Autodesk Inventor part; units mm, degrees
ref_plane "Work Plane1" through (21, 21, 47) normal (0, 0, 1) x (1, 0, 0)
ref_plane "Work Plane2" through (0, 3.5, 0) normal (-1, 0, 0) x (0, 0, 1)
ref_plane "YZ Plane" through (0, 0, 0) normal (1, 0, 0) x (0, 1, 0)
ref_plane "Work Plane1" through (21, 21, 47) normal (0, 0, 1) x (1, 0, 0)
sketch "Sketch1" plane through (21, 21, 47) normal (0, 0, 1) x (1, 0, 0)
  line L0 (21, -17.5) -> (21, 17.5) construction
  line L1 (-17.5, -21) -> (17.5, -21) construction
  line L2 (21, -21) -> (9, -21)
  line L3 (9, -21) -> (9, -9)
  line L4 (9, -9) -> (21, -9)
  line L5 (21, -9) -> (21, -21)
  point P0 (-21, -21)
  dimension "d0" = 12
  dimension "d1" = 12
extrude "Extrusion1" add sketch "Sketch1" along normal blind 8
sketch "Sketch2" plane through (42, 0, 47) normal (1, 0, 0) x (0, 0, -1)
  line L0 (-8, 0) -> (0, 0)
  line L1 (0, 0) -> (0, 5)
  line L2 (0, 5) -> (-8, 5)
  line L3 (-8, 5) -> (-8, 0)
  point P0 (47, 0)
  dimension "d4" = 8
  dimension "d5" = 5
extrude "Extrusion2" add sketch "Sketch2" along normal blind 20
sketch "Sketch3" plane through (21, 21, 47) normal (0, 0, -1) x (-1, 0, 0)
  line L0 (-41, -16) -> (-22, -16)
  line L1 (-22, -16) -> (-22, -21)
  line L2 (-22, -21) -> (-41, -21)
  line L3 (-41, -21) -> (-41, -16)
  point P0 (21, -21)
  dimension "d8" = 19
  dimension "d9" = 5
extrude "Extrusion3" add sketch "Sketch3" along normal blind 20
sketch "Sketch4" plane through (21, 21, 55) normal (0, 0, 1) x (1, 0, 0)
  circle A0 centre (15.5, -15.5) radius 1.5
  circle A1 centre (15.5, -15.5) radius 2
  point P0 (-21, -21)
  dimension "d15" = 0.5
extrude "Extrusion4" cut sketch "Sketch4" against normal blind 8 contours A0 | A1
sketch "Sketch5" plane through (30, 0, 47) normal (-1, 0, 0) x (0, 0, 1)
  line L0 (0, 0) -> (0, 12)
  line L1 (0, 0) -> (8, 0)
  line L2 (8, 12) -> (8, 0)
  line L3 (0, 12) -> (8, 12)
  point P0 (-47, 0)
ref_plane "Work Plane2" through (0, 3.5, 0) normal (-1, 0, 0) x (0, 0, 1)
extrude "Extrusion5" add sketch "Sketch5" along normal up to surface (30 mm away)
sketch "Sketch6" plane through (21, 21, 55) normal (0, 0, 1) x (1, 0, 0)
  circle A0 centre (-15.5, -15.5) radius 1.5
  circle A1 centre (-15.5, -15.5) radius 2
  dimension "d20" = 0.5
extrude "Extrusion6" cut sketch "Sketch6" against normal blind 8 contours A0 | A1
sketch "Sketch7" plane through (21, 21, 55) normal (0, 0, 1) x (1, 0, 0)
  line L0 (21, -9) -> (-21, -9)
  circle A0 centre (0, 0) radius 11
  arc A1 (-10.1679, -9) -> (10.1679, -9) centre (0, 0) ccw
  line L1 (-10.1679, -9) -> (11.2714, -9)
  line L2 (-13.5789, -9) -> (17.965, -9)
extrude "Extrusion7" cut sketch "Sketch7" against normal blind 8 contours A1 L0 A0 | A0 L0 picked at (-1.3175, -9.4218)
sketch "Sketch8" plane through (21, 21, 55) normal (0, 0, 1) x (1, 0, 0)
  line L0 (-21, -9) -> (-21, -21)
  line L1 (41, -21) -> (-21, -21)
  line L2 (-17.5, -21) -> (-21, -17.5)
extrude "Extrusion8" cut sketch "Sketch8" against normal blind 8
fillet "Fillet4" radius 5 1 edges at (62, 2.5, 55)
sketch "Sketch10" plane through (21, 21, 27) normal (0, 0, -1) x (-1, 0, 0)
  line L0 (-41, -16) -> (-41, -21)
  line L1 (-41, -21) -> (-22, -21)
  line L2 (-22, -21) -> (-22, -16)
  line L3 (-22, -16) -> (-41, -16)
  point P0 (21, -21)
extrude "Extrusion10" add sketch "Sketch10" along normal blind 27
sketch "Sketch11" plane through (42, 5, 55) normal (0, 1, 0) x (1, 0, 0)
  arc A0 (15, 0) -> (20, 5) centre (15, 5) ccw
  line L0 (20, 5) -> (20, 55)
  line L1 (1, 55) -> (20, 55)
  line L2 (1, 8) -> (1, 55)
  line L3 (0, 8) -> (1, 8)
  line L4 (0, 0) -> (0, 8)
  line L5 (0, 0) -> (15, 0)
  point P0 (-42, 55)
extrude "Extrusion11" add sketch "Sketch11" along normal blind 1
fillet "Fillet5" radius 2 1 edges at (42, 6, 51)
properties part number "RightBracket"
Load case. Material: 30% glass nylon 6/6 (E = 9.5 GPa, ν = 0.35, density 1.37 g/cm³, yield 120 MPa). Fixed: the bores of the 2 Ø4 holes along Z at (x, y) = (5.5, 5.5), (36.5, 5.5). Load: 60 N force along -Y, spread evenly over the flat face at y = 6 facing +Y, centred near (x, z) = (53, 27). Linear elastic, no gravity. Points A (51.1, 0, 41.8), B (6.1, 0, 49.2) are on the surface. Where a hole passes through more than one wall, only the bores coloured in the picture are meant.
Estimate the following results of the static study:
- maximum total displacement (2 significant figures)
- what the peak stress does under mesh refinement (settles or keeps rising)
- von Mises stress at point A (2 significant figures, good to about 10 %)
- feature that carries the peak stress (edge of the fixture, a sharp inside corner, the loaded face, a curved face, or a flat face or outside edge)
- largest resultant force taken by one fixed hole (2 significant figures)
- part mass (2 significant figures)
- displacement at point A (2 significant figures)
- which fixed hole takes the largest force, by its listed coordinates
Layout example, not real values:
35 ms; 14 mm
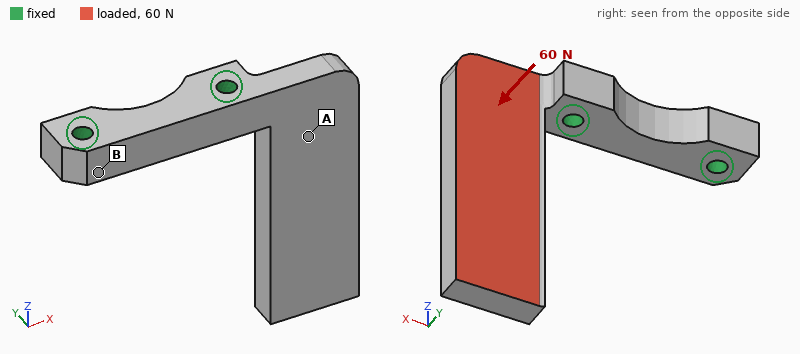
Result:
0.73 mm; keeps rising; 8.7 MPa; a sharp inside corner; 72 N; 13 g; 0.12 mm; (36.5, 5.5)
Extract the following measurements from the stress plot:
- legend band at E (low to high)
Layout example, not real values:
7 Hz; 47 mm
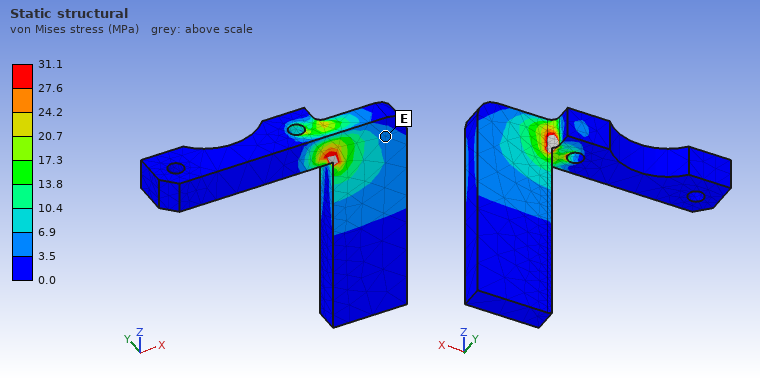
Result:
3.5 to 6.9 MPa
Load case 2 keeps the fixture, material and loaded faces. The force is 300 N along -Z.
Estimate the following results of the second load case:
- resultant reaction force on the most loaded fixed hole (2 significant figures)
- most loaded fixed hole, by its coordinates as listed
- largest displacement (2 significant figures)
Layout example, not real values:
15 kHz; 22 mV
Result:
310 N; (36.5, 5.5); 0.86 mm
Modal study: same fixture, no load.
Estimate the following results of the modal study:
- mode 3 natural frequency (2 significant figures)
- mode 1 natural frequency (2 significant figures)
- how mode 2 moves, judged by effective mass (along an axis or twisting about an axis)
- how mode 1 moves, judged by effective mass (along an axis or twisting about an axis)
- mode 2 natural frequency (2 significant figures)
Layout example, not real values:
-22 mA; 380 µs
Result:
2400 Hz; 630 Hz; along X; along Y; 900 Hz
